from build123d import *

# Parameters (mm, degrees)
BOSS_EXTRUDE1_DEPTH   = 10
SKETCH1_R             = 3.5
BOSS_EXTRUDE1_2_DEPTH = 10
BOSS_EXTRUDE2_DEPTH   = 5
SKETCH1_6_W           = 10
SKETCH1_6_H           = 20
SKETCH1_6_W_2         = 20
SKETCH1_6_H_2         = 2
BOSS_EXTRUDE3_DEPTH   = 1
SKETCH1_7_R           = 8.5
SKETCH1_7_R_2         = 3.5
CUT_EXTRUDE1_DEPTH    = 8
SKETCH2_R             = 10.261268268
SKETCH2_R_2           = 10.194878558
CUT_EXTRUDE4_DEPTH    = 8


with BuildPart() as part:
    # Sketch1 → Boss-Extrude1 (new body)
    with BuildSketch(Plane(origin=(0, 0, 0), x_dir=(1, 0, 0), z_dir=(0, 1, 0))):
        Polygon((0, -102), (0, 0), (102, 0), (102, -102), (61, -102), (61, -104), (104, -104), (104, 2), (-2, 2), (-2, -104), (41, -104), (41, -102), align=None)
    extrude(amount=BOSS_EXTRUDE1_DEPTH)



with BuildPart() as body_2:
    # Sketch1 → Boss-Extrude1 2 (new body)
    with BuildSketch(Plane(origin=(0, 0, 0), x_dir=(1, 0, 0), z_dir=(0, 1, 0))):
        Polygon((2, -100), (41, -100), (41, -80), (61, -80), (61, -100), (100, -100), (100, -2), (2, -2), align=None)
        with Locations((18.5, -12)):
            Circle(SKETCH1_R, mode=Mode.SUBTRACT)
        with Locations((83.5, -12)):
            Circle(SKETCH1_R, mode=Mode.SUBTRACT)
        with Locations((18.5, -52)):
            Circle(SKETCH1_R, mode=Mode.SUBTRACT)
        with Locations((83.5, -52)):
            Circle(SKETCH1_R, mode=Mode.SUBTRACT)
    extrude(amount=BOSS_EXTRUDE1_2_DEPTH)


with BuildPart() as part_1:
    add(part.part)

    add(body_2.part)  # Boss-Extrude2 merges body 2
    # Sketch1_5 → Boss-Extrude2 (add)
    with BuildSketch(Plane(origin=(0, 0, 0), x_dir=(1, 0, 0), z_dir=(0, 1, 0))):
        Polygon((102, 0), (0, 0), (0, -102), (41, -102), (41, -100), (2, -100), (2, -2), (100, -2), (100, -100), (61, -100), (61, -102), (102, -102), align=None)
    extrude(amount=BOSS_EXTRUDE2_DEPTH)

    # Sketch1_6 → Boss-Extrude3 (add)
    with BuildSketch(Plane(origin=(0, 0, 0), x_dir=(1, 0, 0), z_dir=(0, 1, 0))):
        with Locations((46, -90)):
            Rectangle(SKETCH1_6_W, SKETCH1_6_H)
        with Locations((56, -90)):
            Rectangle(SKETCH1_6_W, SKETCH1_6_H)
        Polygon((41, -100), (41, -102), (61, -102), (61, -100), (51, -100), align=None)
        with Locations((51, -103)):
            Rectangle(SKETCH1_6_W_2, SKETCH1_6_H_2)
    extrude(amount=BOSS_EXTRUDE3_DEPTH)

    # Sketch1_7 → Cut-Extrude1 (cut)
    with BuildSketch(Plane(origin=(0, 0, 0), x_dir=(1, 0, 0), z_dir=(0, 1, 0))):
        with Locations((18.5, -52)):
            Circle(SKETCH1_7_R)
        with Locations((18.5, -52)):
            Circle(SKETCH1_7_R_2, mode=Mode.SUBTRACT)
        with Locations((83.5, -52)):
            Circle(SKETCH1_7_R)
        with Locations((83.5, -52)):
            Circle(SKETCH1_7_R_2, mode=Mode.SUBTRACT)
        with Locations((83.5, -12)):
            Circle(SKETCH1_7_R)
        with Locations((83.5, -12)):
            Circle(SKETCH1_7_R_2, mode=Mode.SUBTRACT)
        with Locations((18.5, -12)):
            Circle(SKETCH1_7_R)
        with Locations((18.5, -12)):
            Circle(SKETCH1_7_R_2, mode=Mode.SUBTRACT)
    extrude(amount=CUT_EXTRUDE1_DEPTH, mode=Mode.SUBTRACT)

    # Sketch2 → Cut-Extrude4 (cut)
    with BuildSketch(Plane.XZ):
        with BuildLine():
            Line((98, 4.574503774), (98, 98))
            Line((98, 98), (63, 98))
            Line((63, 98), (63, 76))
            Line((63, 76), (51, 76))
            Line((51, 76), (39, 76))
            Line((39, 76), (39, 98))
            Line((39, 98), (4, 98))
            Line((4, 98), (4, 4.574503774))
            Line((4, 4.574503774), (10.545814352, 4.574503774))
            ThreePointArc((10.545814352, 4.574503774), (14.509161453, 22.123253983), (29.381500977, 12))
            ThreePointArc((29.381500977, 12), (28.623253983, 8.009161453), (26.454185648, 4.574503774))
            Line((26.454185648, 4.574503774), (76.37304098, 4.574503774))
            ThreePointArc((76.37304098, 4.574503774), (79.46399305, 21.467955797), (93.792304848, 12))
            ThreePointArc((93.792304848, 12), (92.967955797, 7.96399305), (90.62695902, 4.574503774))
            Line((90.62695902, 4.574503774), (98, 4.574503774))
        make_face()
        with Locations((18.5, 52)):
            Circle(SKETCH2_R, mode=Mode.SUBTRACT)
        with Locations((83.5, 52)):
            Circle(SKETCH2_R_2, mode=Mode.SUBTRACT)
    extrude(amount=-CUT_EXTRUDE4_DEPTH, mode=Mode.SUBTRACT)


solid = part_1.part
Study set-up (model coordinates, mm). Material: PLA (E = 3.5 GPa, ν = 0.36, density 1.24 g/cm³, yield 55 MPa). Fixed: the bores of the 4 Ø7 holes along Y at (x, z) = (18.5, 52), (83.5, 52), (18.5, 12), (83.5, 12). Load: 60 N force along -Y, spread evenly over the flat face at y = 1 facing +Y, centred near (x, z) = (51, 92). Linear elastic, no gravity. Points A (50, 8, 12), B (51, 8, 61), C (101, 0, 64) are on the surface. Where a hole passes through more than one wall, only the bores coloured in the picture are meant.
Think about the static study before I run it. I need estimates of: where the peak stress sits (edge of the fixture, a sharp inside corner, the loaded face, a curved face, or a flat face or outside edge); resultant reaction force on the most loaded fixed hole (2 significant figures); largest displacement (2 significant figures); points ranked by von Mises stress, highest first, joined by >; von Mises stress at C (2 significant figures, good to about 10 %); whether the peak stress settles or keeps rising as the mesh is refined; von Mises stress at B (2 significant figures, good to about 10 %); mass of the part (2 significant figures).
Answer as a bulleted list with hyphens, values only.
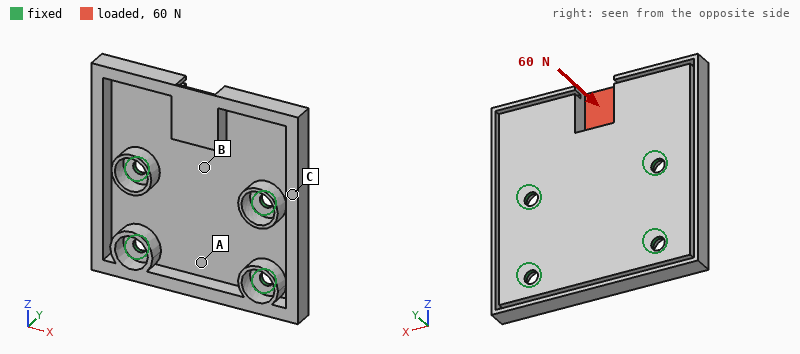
- edge of the fixture
- 80 N
- 1.7 mm
- C > B > A
- 6.7 MPa
- keeps rising
- 4.8 MPa
- 51 g
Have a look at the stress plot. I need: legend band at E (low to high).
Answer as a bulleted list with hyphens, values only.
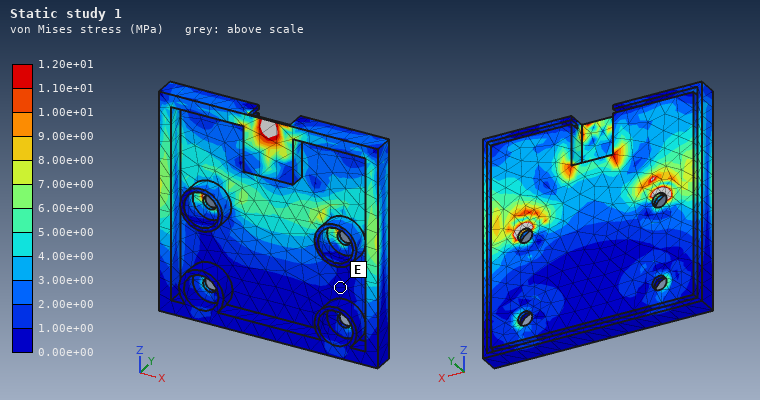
- 0.00e+00 to 1.00e+00 MPa
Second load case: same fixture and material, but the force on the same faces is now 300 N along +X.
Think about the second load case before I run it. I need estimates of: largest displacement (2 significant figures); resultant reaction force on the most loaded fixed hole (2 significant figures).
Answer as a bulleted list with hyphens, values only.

- 0.94 mm
- 220 N
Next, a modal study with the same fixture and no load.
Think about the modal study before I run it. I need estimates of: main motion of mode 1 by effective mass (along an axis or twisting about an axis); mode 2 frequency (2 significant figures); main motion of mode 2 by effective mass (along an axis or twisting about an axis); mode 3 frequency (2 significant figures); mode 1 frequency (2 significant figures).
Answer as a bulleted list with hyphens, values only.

- along Y
- 500 Hz
- twisting about Z
- 900 Hz
- 350 Hz
